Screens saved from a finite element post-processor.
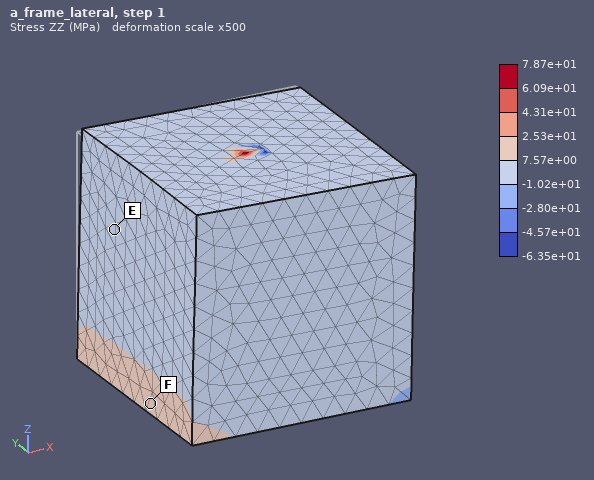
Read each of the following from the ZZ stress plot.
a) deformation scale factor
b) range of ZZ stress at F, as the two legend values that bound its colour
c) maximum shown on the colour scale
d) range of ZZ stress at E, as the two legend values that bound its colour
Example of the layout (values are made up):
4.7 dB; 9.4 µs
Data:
500; 7.57e+00 to 2.53e+01 MPa; 7.87e+01 MPa; -1.02e+01 to 7.57e+00 MPa
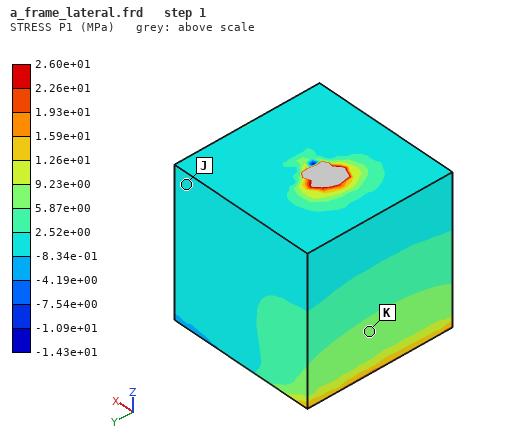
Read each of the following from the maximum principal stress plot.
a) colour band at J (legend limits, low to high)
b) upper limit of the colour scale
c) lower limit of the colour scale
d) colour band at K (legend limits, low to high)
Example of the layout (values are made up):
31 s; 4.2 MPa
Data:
-8.34e-01 to 2.52e+00 MPa; 2.60e+01 MPa; -1.43e+01 MPa; 5.87e+00 to 9.23e+00 MPa
